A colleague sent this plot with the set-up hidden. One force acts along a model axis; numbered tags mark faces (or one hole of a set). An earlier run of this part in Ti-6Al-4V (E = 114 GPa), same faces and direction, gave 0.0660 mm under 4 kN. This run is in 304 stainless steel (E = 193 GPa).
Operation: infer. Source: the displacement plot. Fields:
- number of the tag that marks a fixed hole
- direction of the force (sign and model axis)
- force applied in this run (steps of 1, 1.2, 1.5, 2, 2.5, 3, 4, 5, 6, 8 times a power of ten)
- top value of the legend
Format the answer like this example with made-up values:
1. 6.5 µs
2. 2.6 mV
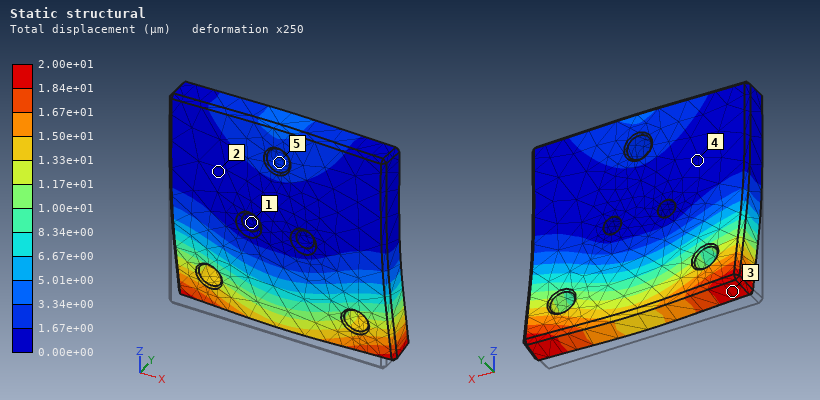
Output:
1. 1
2. +Y
3. 2 kN
4. 2.00e+01 µm
